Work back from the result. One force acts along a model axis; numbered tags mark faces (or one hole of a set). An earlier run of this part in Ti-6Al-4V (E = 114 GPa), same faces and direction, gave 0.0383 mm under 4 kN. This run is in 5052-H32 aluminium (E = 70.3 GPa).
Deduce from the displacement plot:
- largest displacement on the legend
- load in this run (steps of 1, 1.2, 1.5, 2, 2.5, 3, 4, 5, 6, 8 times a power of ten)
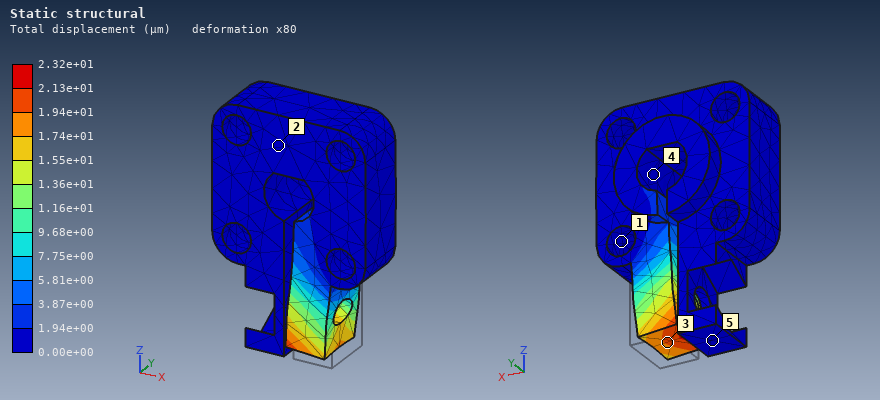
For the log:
2.32e+01 µm
1.5 kN
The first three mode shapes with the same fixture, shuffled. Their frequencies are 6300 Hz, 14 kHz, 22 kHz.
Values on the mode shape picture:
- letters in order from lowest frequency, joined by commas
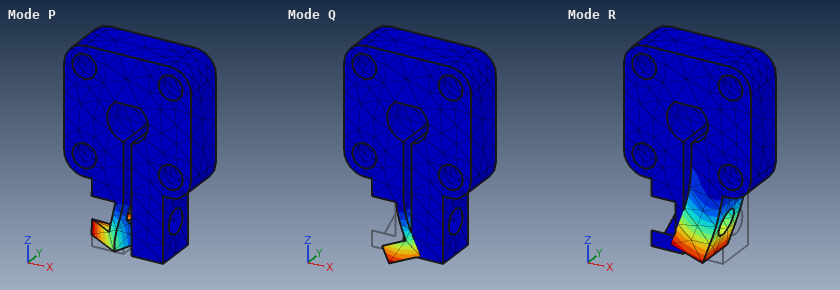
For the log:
Q, P, R
